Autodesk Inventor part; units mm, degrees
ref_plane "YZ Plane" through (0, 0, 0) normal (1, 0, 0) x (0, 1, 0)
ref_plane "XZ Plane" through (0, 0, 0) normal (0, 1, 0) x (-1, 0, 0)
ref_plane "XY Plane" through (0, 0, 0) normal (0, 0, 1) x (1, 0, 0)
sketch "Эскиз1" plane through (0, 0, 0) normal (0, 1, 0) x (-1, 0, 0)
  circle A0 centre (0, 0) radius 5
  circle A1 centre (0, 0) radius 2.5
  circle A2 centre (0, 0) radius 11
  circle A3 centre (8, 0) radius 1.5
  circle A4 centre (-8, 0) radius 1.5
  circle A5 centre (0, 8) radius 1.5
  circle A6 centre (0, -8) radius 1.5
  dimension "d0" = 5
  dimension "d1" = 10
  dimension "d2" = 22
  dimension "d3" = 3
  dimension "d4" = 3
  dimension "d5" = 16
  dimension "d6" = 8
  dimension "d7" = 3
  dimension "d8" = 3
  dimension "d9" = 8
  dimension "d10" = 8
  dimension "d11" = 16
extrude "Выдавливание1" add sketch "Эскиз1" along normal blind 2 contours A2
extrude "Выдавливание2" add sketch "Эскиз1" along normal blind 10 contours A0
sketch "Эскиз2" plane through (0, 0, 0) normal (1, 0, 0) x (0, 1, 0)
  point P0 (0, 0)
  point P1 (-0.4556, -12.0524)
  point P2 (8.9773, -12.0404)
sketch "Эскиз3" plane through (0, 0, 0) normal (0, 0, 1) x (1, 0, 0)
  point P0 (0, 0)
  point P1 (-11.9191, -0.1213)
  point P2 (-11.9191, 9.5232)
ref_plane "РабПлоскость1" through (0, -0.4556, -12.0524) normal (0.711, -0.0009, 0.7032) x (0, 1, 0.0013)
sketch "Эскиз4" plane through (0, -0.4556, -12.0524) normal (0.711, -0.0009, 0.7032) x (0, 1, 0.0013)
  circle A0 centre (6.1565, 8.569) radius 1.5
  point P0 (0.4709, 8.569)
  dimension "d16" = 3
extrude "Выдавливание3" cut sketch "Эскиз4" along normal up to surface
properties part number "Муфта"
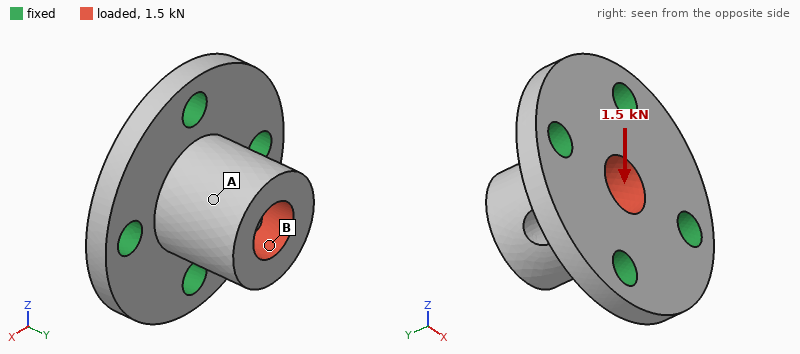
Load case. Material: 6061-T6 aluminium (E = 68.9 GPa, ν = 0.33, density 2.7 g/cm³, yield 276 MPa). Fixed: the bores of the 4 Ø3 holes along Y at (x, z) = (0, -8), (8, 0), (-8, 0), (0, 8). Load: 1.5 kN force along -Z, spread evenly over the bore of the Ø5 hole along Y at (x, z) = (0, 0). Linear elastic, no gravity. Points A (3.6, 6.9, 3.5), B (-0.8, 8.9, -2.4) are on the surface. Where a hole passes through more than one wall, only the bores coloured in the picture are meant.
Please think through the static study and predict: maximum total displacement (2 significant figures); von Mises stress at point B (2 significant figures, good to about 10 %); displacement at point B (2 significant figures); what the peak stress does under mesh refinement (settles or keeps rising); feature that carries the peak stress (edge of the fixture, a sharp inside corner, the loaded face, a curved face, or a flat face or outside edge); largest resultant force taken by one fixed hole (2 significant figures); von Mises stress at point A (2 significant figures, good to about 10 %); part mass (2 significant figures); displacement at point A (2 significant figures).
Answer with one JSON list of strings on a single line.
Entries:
["22 µm", "28 MPa", "19 µm", "keeps rising", "edge of the fixture", "690 N", "15 MPa", "3.0 g", "15 µm"]
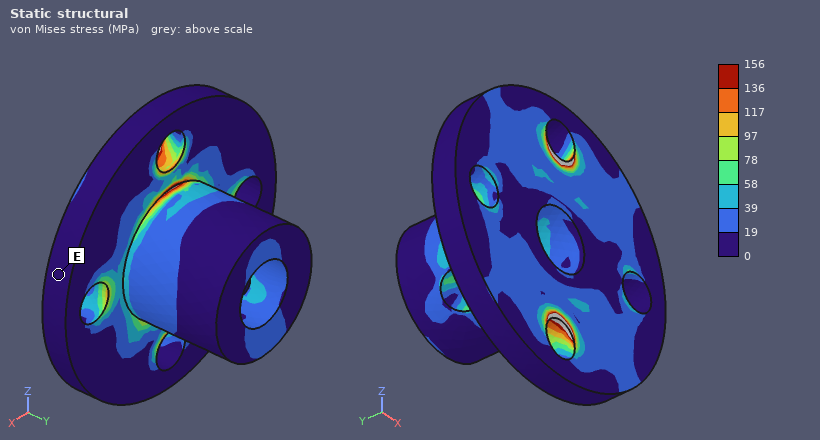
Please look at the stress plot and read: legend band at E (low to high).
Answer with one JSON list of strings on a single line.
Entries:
["0 to 19 MPa"]
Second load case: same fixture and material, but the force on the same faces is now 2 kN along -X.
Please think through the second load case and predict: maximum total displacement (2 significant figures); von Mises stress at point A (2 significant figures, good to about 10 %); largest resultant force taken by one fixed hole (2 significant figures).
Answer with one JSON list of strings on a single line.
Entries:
["30 µm", "20 MPa", "910 N"]
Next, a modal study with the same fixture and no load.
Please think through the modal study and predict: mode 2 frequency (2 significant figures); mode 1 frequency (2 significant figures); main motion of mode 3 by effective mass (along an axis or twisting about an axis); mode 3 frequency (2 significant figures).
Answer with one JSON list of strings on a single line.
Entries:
["39 kHz", "38 kHz", "along Y", "55 kHz"]
